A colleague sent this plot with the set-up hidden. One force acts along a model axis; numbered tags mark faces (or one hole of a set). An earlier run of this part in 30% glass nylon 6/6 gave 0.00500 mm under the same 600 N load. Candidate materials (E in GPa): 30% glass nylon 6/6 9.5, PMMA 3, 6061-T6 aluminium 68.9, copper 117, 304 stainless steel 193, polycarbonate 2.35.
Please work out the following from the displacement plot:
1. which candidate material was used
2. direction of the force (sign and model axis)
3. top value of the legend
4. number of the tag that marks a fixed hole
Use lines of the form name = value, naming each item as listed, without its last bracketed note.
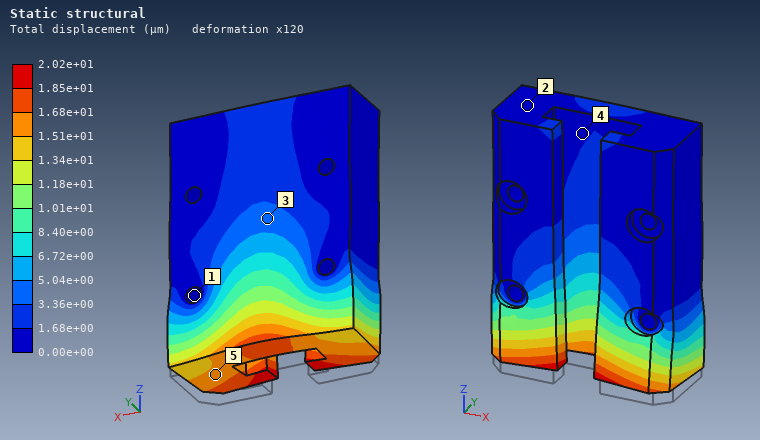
which candidate material was used = polycarbonate
direction of the force = +Z
top value of the legend = 2.02e+01 µm
number of the tag that marks a fixed hole = 1
